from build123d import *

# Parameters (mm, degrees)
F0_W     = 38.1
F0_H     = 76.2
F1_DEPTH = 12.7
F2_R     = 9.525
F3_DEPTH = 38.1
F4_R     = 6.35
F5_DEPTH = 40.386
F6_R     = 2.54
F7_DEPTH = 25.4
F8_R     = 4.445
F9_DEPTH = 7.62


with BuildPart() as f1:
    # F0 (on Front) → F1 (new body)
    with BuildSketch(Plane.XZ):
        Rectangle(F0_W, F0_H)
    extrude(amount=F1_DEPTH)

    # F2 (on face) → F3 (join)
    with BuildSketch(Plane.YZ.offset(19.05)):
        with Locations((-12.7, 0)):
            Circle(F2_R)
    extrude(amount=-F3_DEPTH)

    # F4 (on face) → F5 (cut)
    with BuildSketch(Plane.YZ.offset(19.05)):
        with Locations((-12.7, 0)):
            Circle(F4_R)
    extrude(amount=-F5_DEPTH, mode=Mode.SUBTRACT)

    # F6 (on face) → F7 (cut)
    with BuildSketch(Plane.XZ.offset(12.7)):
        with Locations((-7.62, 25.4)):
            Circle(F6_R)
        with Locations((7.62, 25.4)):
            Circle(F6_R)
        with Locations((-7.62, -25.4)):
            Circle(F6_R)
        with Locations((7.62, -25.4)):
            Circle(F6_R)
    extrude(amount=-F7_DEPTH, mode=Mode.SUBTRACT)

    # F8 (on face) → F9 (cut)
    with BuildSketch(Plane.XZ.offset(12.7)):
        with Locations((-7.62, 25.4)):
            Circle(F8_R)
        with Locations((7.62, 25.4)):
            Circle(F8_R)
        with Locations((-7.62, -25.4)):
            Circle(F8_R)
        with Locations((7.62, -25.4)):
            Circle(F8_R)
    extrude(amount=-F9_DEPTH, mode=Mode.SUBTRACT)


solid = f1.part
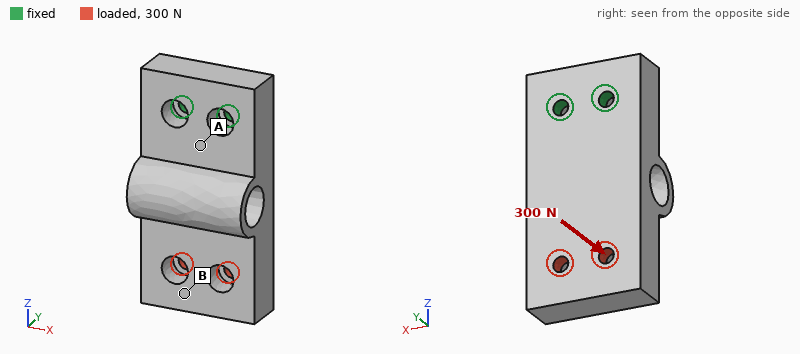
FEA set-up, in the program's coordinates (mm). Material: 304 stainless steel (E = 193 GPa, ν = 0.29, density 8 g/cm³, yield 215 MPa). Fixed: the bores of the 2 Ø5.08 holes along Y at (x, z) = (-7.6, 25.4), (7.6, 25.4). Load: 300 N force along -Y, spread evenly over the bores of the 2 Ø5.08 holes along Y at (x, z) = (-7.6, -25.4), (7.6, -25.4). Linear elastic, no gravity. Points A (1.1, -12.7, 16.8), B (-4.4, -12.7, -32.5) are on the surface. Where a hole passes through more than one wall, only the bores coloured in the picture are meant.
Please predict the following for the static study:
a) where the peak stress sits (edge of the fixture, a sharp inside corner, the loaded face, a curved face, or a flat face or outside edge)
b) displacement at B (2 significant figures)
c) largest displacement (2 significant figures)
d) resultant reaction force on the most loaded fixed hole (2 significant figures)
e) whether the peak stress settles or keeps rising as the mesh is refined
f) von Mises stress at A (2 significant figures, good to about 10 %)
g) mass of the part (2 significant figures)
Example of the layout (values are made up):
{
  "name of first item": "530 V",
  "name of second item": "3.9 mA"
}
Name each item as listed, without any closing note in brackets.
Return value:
{
  "where the peak stress sits": "edge of the fixture",
  "displacement at B": "37 µm",
  "largest displacement": "41 µm",
  "resultant reaction force on the most loaded fixed hole": "160 N",
  "whether the peak stress settles or keeps rising as the mesh is refined": "keeps rising",
  "von Mises stress at A": "15 MPa",
  "mass of the part": "280 g"
}
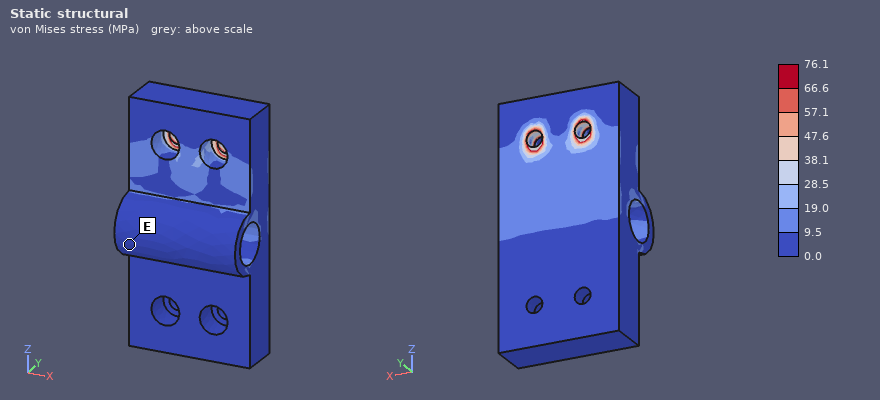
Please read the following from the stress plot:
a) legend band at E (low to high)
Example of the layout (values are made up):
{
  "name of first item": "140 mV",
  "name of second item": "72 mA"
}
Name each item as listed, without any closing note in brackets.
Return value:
{
  "legend band at E": "0.0 to 9.5 MPa"
}
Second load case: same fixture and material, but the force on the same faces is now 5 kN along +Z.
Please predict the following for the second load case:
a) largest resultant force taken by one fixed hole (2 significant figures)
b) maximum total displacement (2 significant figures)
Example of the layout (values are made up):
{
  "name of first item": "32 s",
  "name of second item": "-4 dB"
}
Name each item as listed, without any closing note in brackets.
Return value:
{
  "largest resultant force taken by one fixed hole": "2.5 kN",
  "maximum total displacement": "26 µm"
}
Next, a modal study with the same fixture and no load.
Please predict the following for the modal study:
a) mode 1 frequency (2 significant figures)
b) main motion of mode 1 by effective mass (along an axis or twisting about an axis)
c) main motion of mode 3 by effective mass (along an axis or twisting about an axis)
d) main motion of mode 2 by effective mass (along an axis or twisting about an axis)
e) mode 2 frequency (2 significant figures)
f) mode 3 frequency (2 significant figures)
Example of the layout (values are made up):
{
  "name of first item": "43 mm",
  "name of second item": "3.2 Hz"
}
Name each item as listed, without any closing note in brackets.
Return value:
{
  "mode 1 frequency": "1500 Hz",
  "main motion of mode 1 by effective mass": "along Y",
  "main motion of mode 3 by effective mass": "twisting about Z",
  "main motion of mode 2 by effective mass": "along X",
  "mode 2 frequency": "3900 Hz",
  "mode 3 frequency": "6500 Hz"
}
